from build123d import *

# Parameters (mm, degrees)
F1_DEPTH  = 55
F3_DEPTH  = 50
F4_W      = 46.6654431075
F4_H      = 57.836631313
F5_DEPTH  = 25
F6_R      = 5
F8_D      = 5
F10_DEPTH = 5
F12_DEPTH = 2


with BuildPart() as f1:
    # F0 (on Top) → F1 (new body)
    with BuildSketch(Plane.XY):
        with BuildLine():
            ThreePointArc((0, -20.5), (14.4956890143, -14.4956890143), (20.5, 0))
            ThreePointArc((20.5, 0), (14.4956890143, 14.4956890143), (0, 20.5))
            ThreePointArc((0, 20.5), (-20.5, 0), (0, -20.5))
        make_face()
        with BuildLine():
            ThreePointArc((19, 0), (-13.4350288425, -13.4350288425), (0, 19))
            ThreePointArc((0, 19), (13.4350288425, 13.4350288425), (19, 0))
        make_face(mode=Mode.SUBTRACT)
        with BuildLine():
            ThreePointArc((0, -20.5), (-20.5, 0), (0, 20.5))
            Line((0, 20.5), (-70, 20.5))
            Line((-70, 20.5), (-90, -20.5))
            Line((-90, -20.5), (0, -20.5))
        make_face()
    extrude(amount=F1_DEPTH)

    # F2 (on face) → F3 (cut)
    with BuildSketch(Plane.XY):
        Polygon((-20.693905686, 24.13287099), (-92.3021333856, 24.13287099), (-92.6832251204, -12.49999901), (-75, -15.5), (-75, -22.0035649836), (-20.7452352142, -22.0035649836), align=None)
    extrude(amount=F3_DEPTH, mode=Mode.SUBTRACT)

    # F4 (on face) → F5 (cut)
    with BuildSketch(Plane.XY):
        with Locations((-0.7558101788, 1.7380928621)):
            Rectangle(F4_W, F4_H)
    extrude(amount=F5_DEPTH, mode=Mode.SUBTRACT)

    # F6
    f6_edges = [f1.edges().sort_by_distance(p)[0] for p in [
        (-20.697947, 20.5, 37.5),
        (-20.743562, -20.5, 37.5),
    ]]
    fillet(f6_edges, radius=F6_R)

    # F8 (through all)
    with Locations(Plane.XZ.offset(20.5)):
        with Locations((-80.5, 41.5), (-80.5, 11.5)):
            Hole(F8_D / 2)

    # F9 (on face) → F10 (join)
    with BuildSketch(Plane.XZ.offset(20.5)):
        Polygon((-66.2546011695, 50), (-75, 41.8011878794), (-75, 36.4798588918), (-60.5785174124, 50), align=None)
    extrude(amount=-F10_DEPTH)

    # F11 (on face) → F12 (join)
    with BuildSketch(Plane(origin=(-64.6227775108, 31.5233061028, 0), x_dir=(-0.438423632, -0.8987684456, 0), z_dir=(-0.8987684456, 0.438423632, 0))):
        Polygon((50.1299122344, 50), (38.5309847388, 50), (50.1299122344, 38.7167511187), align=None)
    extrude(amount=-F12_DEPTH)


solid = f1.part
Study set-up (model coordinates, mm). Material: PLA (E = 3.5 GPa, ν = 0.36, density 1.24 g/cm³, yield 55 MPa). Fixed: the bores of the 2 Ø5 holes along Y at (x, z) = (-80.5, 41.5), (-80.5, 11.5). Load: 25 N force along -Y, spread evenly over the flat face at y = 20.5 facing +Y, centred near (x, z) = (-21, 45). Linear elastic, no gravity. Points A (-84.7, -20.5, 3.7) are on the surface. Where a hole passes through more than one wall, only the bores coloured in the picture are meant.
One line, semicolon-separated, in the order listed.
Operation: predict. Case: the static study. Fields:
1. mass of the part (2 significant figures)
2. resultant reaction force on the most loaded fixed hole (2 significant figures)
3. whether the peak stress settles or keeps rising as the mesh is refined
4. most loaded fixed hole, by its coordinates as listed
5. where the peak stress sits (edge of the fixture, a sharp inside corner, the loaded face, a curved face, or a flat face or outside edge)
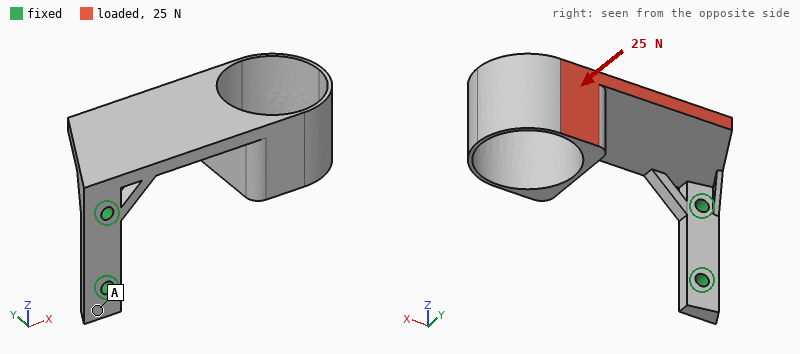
34 g; 26 N; keeps rising; (-80.5, 41.5); edge of the fixture
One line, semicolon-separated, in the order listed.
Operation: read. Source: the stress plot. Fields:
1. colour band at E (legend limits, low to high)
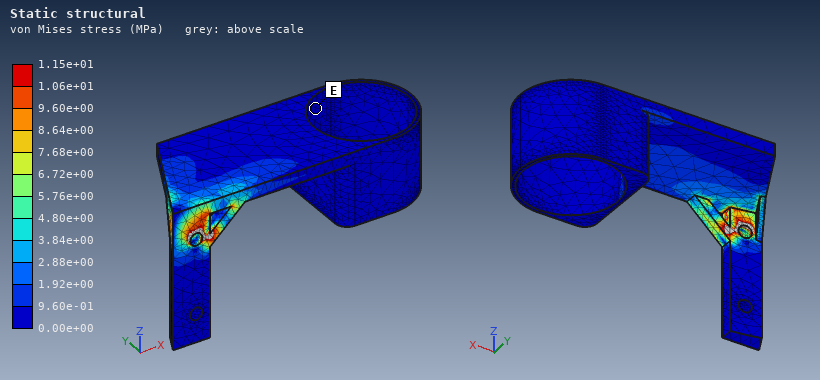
0.00e+00 to 9.60e-01 MPa
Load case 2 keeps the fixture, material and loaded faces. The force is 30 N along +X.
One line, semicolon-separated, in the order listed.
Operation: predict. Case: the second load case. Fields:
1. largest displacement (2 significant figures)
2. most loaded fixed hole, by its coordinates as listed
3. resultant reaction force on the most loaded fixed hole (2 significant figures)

1.3 mm; (-80.5, 41.5); 32 N
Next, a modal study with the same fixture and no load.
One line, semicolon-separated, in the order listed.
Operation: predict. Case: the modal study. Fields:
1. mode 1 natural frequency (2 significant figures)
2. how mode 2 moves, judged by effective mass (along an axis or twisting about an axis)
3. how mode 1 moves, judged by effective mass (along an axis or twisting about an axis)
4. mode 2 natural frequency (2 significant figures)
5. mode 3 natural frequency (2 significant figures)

120 Hz; along Y; along Z; 170 Hz; 350 Hz
